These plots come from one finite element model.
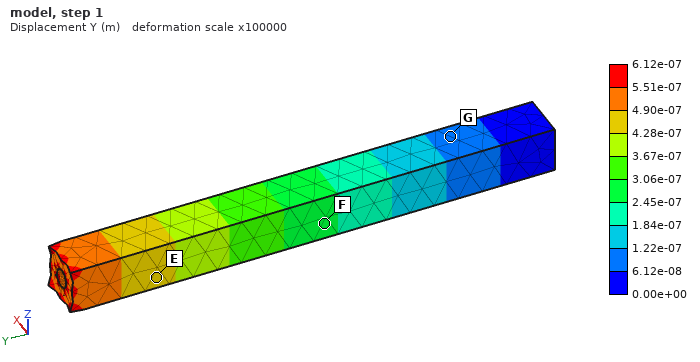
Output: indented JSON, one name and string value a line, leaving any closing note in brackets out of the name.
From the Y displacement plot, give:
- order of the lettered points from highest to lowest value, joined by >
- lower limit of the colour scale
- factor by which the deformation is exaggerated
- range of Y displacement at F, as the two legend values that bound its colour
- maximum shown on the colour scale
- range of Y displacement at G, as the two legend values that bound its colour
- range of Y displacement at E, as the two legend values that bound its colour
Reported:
{
  "order of the lettered points from highest to lowest value, joined by >": "E > F > G",
  "lower limit of the colour scale": "0.00e+00 m",
  "factor by which the deformation is exaggerated": "100000",
  "range of Y displacement at F, as the two legend values that bound its colour": "2.45e-07 to 3.06e-07 m",
  "maximum shown on the colour scale": "6.12e-07 m",
  "range of Y displacement at G, as the two legend values that bound its colour": "6.12e-08 to 1.22e-07 m",
  "range of Y displacement at E, as the two legend values that bound its colour": "4.28e-07 to 4.90e-07 m"
}
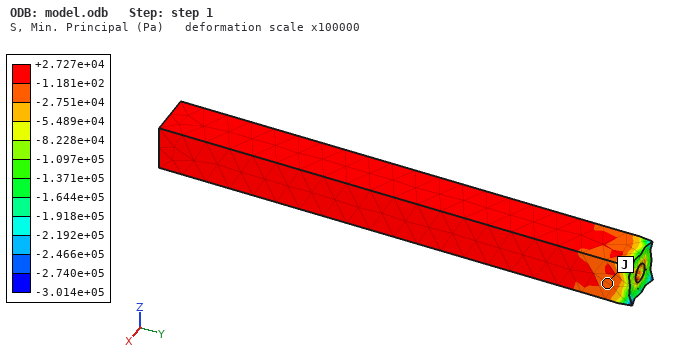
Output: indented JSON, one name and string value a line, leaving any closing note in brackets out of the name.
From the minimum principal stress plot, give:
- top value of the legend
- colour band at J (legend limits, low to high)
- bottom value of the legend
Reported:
{
  "top value of the legend": "+2.727e+04 Pa",
  "colour band at J": "-2.751e+04 to -1.181e+02 Pa",
  "bottom value of the legend": "-3.014e+05 Pa"
}
